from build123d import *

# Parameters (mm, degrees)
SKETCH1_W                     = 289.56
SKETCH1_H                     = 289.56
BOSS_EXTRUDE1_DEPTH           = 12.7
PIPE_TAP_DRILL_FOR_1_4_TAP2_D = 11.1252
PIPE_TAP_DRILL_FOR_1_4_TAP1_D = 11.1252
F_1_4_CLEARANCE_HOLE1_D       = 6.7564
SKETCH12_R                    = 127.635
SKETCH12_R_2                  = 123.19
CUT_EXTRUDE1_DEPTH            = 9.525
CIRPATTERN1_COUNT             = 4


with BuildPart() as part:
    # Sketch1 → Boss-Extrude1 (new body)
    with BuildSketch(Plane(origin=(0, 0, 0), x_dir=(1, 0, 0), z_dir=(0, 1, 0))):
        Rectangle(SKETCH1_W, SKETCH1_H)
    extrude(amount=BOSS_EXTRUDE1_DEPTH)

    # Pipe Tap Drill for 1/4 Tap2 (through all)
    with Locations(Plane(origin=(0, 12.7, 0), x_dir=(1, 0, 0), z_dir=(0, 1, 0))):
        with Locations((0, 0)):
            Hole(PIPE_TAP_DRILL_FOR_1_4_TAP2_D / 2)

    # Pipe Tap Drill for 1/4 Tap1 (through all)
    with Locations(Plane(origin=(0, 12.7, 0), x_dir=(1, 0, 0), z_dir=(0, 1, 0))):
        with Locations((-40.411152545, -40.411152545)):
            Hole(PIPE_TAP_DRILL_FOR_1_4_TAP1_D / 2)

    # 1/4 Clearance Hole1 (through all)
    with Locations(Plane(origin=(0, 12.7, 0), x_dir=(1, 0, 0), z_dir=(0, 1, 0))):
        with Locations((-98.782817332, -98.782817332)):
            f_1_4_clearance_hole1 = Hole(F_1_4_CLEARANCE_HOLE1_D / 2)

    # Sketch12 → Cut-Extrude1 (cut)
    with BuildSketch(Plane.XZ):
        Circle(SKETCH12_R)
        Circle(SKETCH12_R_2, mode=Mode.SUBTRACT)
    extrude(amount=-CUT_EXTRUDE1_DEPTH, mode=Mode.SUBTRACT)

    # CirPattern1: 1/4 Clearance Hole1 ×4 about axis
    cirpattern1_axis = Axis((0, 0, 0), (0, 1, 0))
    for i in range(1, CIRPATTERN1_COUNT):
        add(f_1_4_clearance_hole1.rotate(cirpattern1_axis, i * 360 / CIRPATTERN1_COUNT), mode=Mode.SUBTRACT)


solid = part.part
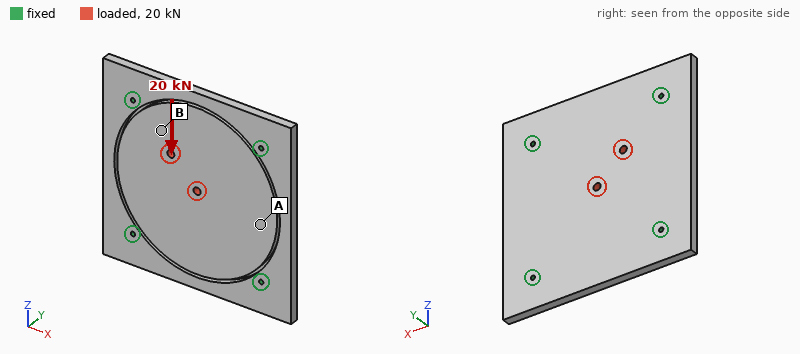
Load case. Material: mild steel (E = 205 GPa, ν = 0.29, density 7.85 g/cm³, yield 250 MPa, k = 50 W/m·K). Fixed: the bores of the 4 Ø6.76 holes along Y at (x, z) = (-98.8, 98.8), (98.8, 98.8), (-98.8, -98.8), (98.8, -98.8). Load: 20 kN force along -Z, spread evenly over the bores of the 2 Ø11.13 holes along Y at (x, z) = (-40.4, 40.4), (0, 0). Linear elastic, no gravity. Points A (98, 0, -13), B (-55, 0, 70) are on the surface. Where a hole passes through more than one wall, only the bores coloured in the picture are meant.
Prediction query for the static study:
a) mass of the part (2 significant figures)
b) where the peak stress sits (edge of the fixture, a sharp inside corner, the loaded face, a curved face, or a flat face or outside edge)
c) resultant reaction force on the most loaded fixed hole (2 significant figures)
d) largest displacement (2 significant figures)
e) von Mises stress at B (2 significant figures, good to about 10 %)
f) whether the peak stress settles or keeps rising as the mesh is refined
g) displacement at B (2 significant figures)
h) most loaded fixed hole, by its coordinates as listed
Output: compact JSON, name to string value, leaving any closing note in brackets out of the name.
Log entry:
{"mass of the part": "8.1 kg", "where the peak stress sits": "edge of the fixture", "resultant reaction force on the most loaded fixed hole": "6.2 kN", "largest displacement": "8.8 µm", "von Mises stress at B": "7.8 MPa", "whether the peak stress settles or keeps rising as the mesh is refined": "keeps rising", "displacement at B": "6.3 µm", "most loaded fixed hole, by its coordinates as listed": "(-98.8, 98.8)"}
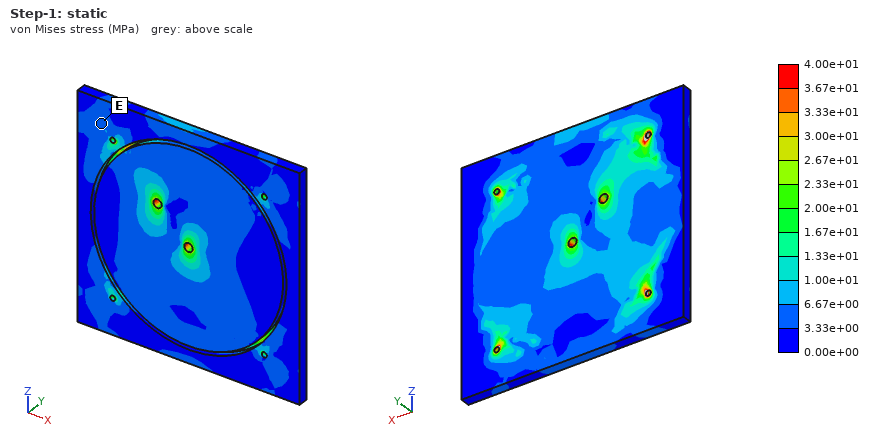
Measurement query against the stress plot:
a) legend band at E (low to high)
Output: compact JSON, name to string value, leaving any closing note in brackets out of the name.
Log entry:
{"legend band at E": "3.33e+00 to 6.67e+00 MPa"}
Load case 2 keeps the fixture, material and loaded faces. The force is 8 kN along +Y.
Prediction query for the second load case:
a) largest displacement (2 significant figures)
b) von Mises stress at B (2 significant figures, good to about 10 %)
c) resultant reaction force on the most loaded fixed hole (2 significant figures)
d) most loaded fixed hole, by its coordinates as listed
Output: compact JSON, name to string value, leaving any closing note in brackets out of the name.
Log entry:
{"largest displacement": "0.14 mm", "von Mises stress at B": "26 MPa", "resultant reaction force on the most loaded fixed hole": "5.5 kN", "most loaded fixed hole, by its coordinates as listed": "(-98.8, 98.8)"}
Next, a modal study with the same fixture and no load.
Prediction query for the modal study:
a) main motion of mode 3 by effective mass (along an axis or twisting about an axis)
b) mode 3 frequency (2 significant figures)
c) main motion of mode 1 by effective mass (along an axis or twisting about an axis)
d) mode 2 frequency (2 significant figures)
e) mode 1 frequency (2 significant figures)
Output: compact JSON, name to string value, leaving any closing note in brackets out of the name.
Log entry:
{"main motion of mode 3 by effective mass": "twisting about X", "mode 3 frequency": "1400 Hz", "main motion of mode 1 by effective mass": "along Y", "mode 2 frequency": "1400 Hz", "mode 1 frequency": "920 Hz"}
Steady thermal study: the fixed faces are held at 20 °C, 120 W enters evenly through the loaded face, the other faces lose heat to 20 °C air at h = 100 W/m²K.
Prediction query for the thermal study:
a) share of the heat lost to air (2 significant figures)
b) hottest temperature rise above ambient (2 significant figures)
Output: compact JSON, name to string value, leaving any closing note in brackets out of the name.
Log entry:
{"share of the heat lost to air": "91 %", "hottest temperature rise above ambient": "46 K"}
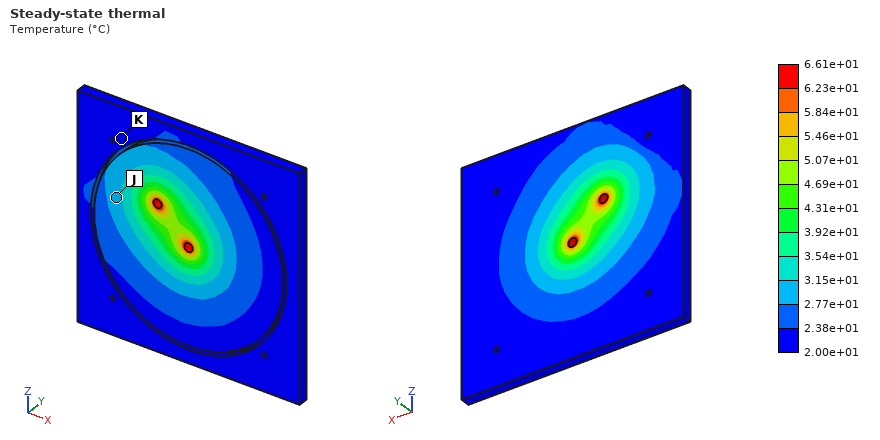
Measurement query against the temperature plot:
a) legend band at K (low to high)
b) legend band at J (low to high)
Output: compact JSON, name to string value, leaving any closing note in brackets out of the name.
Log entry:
{"legend band at K": "2.00e+01 to 2.38e+01 °C", "legend band at J": "2.77e+01 to 3.15e+01 °C"}
